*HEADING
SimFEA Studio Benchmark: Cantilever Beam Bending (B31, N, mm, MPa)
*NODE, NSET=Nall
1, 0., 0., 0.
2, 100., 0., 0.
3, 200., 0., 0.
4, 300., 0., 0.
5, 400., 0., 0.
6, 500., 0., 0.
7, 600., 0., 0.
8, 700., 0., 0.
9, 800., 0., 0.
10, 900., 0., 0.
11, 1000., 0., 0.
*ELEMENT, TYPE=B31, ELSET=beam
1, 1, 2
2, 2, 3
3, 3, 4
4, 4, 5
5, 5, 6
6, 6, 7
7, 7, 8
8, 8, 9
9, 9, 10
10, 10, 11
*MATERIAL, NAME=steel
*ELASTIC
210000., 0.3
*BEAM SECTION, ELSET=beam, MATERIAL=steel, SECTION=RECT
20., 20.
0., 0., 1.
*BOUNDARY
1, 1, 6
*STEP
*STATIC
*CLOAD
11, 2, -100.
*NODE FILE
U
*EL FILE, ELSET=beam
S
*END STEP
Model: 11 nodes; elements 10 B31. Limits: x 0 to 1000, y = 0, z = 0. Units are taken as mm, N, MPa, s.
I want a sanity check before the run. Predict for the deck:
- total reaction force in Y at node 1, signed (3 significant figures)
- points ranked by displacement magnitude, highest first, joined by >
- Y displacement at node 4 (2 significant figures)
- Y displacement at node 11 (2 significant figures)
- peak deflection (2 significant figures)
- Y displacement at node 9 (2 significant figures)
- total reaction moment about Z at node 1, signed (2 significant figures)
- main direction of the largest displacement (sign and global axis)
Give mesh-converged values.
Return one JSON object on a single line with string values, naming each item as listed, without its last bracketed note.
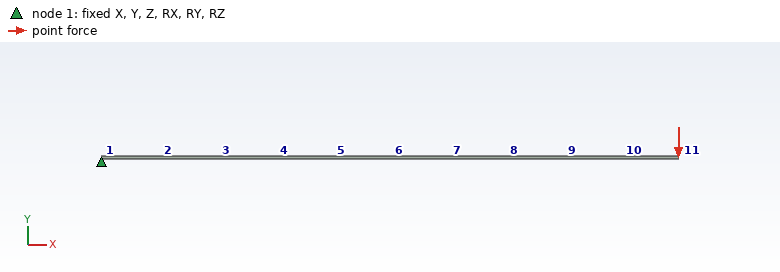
{"total reaction force in Y at node 1, signed": "100 N", "points ranked by displacement magnitude, highest first, joined by >": "node 11 > node 10 > node 9 > node 4 > node 1", "Y displacement at node 4": "-1.4 mm", "Y displacement at node 11": "-12 mm", "peak deflection": "12 mm", "Y displacement at node 9": "-8.4 mm", "total reaction moment about Z at node 1, signed": "100000 N·mm", "main direction of the largest displacement": "-Y"}
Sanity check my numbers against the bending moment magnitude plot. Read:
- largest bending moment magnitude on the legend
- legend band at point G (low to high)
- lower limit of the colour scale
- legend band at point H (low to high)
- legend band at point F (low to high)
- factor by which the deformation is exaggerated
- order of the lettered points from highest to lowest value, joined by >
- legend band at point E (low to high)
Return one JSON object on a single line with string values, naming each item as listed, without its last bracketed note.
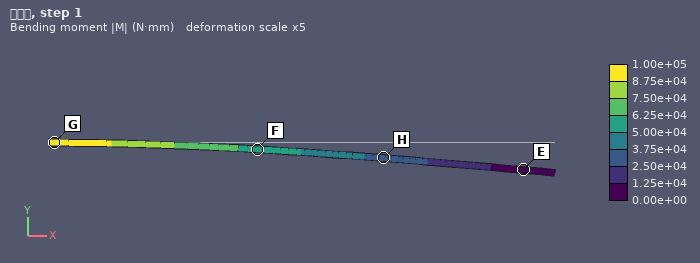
{"largest bending moment magnitude on the legend": "1.00e+05 N·mm", "legend band at point G": "8.75e+04 to 1.00e+05 N·mm", "lower limit of the colour scale": "0.00e+00 N·mm", "legend band at point H": "2.50e+04 to 3.75e+04 N·mm", "legend band at point F": "5.00e+04 to 6.25e+04 N·mm", "factor by which the deformation is exaggerated": "5", "order of the lettered points from highest to lowest value, joined by >": "G > F > H > E", "legend band at point E": "0.00e+00 to 1.25e+04 N·mm"}
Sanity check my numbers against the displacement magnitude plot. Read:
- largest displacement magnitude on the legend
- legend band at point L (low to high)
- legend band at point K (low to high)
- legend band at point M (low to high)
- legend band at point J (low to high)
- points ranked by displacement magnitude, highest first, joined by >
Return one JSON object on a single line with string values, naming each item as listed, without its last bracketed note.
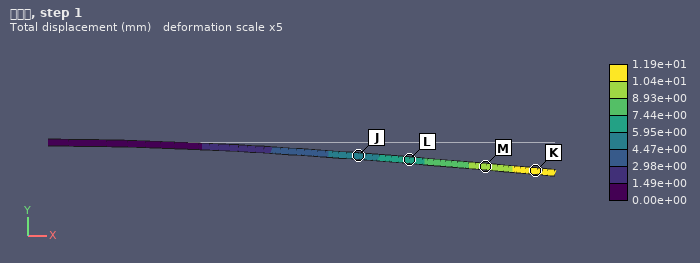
{"largest displacement magnitude on the legend": "1.19e+01 mm", "legend band at point L": "5.95e+00 to 7.44e+00 mm", "legend band at point K": "1.04e+01 to 1.19e+01 mm", "legend band at point M": "8.93e+00 to 1.04e+01 mm", "legend band at point J": "4.47e+00 to 5.95e+00 mm", "points ranked by displacement magnitude, highest first, joined by >": "K > M > L > J"}
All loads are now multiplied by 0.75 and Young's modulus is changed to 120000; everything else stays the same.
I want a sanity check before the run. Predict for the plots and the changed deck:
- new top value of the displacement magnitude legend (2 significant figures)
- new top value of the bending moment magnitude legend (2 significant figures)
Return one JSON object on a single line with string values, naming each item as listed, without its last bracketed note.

{"new top value of the displacement magnitude legend": "16 mm", "new top value of the bending moment magnitude legend": "75000 N·mm"}
